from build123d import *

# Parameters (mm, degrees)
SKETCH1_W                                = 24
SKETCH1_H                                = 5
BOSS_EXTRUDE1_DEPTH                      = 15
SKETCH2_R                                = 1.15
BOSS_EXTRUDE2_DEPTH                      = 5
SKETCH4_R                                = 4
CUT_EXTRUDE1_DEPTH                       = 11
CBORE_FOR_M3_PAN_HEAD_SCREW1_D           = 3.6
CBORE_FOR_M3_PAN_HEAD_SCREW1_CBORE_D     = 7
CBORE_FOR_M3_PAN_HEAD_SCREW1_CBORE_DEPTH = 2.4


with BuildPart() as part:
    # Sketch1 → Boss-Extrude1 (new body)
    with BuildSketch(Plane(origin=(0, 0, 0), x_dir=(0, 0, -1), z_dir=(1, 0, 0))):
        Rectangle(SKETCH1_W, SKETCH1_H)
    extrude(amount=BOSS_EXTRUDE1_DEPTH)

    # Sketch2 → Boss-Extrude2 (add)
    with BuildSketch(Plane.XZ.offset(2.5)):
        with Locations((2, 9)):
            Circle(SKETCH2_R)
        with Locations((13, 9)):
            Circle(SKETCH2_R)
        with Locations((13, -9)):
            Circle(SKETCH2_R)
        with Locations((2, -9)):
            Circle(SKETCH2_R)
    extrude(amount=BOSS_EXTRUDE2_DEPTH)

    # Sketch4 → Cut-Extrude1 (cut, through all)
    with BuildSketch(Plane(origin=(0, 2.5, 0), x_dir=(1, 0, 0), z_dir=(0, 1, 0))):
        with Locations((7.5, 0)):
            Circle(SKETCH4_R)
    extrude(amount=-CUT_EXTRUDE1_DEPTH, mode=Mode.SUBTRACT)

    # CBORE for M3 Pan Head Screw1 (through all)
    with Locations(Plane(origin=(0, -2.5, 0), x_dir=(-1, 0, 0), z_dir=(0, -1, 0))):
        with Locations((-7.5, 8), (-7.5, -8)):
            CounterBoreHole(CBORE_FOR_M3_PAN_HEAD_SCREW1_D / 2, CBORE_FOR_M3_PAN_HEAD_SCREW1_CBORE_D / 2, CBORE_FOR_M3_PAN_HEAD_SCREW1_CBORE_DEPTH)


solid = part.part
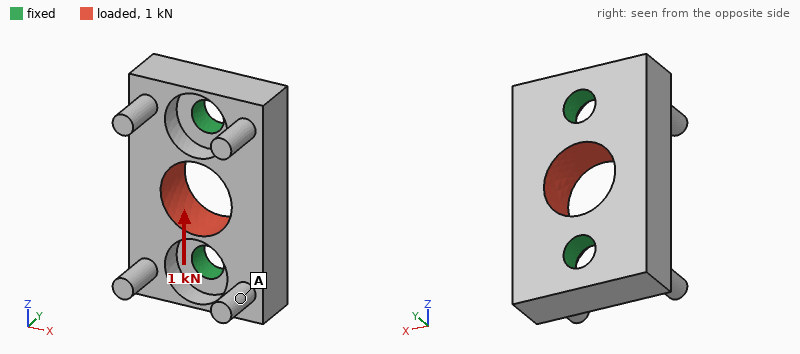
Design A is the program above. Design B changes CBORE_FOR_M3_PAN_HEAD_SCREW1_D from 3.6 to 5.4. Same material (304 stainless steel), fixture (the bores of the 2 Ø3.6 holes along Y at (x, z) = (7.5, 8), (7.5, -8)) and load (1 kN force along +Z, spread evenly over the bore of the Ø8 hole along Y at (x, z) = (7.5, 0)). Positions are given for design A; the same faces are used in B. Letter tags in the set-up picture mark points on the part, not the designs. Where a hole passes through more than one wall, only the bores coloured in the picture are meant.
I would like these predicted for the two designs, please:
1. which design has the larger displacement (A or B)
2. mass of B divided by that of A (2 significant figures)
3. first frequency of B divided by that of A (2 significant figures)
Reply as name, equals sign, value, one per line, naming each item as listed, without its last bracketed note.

which design has the larger displacement = A
mass of B divided by that of A = 0.95
first frequency of B divided by that of A = 1.4
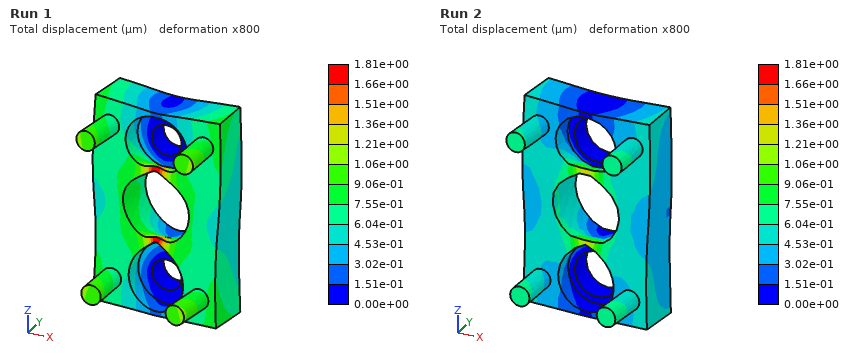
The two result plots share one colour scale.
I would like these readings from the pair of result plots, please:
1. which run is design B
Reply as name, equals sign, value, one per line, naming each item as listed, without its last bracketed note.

which run is design B = Run 2
